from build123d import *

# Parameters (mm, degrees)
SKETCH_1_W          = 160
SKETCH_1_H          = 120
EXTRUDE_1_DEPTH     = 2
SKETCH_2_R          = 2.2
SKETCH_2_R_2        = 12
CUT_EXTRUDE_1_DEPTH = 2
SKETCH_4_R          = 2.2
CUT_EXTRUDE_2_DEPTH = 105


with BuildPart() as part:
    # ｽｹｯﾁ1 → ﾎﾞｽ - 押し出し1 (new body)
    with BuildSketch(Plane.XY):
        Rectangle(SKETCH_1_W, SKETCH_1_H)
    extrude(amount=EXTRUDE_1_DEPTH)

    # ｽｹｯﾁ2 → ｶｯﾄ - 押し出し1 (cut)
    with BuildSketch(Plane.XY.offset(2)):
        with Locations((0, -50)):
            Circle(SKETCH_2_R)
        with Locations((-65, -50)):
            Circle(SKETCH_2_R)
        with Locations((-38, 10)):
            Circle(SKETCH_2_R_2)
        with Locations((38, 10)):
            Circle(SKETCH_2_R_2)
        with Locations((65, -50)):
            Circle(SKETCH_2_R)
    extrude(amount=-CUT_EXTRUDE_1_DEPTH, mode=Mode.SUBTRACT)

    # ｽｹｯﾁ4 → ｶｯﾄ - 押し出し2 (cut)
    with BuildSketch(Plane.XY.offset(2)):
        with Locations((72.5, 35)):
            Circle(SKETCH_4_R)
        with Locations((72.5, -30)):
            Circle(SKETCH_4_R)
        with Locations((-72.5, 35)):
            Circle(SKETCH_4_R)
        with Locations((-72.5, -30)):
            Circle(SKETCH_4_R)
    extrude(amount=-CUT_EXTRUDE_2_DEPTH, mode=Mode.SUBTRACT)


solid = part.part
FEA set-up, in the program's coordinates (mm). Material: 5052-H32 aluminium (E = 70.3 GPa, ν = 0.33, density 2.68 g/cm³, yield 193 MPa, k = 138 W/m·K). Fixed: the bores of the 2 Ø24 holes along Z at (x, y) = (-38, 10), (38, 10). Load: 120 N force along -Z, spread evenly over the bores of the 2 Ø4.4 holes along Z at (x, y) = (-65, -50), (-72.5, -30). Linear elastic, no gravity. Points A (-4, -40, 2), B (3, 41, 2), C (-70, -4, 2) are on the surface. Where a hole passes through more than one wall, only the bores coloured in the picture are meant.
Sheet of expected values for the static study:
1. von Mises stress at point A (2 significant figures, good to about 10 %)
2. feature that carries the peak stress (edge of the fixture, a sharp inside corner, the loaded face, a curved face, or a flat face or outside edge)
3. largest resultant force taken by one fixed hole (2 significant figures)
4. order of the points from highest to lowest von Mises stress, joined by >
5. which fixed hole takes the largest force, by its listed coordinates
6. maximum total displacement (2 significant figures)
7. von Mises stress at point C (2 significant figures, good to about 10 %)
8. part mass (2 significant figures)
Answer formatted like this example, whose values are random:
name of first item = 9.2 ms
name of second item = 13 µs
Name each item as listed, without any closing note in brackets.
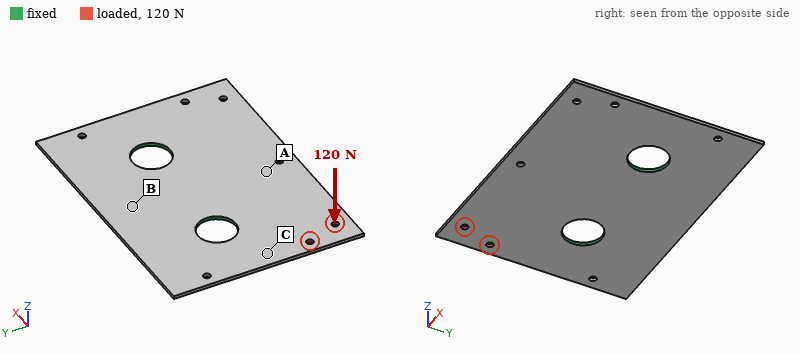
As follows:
von Mises stress at point A = 30 MPa
feature that carries the peak stress = a flat face or outside edge
largest resultant force taken by one fixed hole = 130 N
order of the points from highest to lowest von Mises stress, joined by > = C > A > B
which fixed hole takes the largest force, by its listed coordinates = (-38, 10)
maximum total displacement = 2.2 mm
von Mises stress at point C = 68 MPa
part mass = 97 g
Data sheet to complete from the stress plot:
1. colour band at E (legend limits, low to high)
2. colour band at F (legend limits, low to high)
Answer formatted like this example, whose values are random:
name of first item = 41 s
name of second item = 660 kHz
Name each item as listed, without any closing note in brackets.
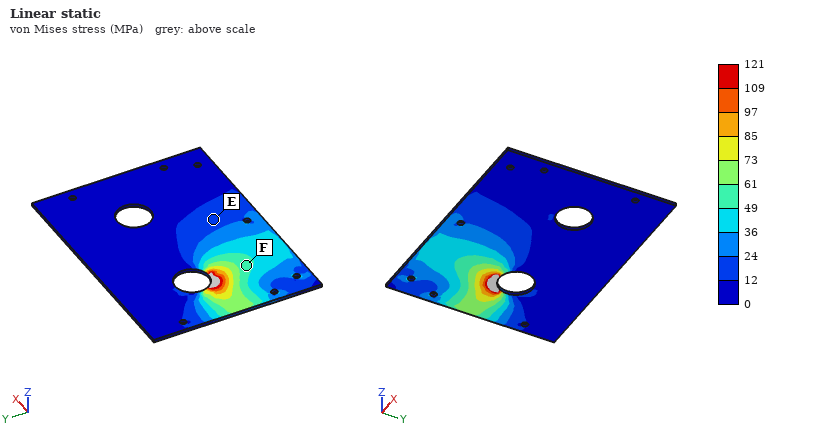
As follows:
colour band at E = 12 to 24 MPa
colour band at F = 49 to 61 MPa
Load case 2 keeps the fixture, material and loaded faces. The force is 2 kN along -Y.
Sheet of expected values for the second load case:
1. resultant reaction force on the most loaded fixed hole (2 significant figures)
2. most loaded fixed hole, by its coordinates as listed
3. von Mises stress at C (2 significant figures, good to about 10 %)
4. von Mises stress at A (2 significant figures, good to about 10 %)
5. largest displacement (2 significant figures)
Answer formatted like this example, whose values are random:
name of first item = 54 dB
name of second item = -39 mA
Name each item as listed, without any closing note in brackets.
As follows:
resultant reaction force on the most loaded fixed hole = 2.5 kN
most loaded fixed hole, by its coordinates as listed = (-38, 10)
von Mises stress at C = 22 MPa
von Mises stress at A = 7.5 MPa
largest displacement = 39 µm
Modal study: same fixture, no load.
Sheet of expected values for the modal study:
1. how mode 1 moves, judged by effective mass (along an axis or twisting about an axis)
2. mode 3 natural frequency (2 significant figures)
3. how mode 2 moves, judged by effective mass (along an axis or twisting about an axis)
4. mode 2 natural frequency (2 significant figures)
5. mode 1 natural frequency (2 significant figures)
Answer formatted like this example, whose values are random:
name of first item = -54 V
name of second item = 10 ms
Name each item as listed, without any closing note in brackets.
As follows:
how mode 1 moves, judged by effective mass = along Z
mode 3 natural frequency = 820 Hz
how mode 2 moves, judged by effective mass = twisting about Y
mode 2 natural frequency = 540 Hz
mode 1 natural frequency = 430 Hz
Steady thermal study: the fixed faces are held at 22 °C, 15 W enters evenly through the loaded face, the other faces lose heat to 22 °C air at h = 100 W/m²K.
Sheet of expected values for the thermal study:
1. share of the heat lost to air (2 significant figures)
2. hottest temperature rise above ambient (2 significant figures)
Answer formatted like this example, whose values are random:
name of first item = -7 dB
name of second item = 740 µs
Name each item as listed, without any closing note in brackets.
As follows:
share of the heat lost to air = 68 %
hottest temperature rise above ambient = 30 K
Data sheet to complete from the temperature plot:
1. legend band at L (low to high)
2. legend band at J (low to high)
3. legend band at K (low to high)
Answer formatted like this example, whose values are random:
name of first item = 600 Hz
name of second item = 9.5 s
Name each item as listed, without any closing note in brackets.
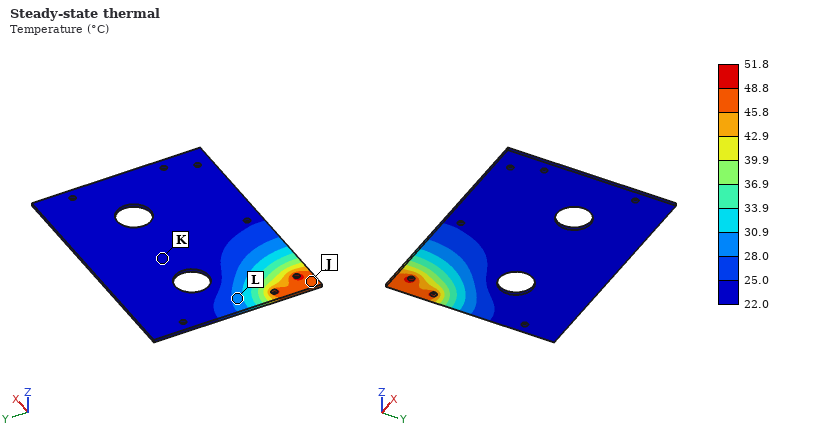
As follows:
legend band at L = 28.0 to 30.9 °C
legend band at J = 45.8 to 48.8 °C
legend band at K = 22.0 to 25.0 °C
